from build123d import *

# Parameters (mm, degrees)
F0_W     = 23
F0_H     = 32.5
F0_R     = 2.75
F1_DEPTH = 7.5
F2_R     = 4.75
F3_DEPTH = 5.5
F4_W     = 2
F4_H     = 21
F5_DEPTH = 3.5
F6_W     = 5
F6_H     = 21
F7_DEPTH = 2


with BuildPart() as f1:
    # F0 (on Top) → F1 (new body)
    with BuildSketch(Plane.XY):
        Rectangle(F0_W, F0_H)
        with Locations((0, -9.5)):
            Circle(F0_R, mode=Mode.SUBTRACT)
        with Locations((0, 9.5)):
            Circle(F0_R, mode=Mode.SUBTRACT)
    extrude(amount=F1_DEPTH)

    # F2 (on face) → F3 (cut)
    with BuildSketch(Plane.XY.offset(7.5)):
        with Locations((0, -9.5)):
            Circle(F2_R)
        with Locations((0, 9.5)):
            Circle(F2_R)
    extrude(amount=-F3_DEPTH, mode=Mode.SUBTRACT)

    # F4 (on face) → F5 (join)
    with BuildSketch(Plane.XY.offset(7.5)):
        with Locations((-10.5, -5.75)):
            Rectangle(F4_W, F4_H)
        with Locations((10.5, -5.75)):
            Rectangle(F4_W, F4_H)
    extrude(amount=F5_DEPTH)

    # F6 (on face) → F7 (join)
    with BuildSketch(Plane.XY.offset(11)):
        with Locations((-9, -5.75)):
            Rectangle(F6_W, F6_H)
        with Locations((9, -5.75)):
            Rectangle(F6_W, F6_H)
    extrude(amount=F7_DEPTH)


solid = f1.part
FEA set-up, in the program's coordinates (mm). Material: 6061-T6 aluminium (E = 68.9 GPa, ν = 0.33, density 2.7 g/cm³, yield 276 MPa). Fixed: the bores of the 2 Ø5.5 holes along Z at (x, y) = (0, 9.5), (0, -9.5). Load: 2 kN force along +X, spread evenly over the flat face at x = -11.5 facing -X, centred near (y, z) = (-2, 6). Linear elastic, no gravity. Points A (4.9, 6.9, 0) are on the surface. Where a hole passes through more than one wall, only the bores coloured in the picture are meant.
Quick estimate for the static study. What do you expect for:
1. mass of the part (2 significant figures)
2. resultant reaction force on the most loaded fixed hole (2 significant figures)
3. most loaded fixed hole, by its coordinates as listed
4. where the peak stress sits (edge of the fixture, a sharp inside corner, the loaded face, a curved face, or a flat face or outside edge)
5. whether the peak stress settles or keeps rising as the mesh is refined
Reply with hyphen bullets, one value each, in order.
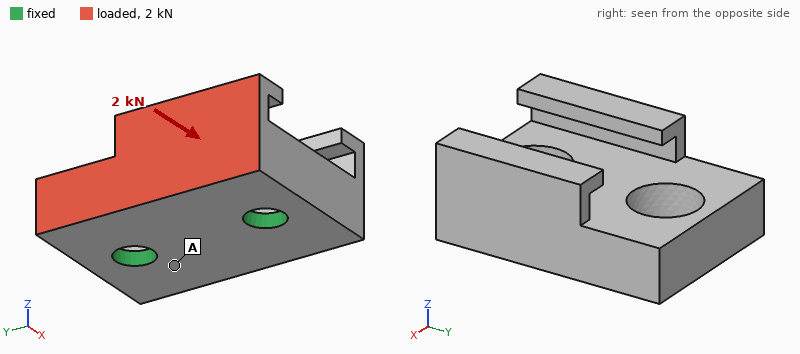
- 15 g
- 1.2 kN
- (0, -9.5)
- edge of the fixture
- keeps rising
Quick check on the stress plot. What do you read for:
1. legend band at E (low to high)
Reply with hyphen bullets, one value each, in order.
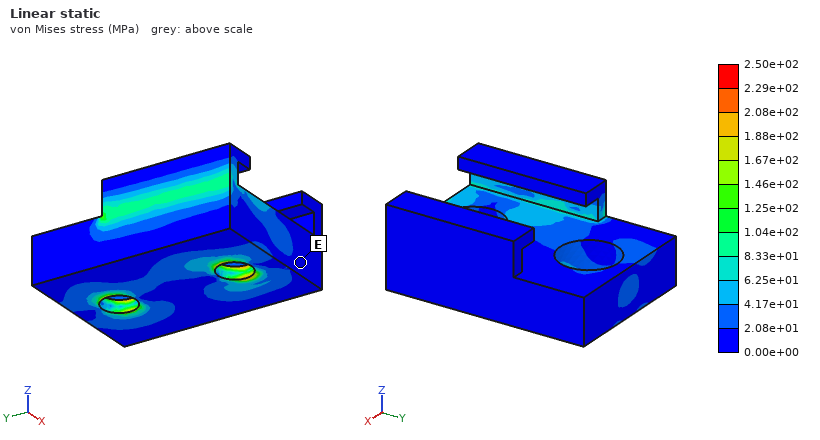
- 0.00e+00 to 2.08e+01 MPa
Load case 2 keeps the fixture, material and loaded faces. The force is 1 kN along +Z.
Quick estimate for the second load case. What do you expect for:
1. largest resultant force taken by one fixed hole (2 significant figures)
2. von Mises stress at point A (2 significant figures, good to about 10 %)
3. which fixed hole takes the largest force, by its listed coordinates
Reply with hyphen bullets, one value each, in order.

- 600 N
- 24 MPa
- (0, -9.5)
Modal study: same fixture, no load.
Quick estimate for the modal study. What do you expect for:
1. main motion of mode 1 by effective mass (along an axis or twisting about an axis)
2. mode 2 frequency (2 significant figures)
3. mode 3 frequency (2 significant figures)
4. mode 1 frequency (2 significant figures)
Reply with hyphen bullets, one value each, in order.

- along X
- 20 kHz
- 20 kHz
- 8800 Hz
